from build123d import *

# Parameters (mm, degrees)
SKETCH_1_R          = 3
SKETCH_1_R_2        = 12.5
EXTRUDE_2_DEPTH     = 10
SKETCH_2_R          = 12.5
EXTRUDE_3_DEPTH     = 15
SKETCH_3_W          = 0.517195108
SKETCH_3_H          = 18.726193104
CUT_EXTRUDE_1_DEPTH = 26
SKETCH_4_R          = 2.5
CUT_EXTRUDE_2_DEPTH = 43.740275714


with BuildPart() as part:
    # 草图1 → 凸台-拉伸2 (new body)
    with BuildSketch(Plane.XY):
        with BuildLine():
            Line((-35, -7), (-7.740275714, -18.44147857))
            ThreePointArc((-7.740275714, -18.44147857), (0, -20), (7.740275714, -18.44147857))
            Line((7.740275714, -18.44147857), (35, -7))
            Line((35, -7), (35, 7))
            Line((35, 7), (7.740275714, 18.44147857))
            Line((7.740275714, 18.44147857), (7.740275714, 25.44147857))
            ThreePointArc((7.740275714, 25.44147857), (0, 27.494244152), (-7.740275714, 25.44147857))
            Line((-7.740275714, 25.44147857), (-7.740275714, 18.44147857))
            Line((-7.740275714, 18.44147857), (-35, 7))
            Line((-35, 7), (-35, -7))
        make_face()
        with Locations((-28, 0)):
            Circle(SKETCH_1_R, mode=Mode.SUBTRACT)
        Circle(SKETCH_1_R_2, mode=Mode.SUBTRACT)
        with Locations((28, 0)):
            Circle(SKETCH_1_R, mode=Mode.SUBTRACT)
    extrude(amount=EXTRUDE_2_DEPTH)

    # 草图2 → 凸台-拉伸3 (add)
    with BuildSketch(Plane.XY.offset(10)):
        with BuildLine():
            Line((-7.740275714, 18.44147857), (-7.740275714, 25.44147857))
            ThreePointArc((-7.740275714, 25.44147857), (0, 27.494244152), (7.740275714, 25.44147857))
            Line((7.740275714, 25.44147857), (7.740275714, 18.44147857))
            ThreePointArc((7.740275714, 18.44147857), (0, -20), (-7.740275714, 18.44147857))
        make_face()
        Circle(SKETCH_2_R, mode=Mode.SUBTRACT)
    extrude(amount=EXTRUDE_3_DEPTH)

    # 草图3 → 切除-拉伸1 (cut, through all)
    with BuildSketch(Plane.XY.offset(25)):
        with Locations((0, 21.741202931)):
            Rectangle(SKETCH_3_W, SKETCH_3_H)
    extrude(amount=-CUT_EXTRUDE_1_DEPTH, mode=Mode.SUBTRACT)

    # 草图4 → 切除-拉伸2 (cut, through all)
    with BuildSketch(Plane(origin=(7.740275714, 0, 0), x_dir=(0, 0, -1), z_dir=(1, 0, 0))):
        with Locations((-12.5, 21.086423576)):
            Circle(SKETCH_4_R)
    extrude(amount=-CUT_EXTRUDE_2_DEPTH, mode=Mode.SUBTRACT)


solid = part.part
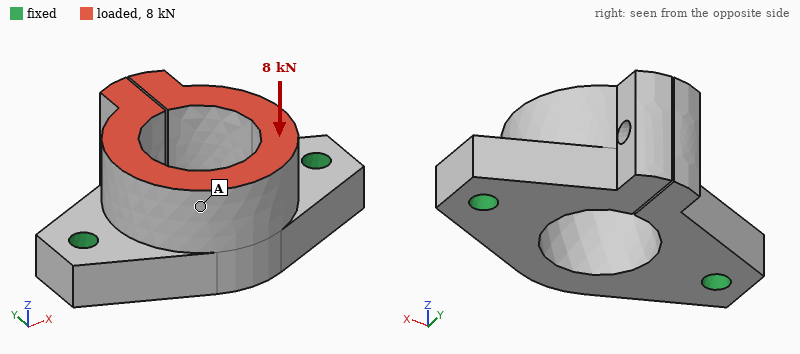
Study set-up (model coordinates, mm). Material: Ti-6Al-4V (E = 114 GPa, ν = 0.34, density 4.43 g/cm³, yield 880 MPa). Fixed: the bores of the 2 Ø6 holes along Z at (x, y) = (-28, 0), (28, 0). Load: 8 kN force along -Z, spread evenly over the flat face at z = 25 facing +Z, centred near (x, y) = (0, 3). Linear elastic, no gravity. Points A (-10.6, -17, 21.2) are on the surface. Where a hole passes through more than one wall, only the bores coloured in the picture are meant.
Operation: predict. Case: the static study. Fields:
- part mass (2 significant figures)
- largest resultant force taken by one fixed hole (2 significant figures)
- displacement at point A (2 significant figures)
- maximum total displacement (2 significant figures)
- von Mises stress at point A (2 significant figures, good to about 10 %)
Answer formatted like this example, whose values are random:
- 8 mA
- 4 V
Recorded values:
- 130 g
- 4.0 kN
- 15 µm
- 88 µm
- 38 MPa
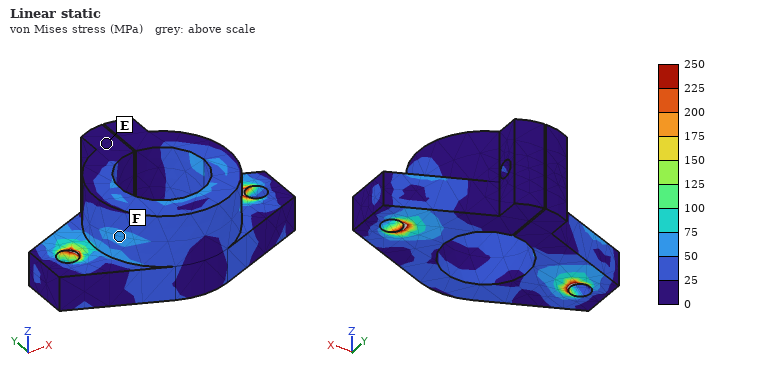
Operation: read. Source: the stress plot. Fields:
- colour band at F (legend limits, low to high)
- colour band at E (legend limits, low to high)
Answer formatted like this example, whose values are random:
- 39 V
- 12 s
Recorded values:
- 50 to 75 MPa
- 0 to 25 MPa
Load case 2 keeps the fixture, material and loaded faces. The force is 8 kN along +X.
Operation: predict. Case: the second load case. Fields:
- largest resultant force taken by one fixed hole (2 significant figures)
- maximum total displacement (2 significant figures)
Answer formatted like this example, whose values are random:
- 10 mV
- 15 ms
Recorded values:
- 4.5 kN
- 0.16 mm
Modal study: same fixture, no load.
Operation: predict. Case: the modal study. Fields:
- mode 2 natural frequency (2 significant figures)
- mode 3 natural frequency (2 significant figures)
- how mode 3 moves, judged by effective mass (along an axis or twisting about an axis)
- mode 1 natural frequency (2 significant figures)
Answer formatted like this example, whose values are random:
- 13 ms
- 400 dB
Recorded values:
- 5600 Hz
- 6100 Hz
- along Y
- 5500 Hz
